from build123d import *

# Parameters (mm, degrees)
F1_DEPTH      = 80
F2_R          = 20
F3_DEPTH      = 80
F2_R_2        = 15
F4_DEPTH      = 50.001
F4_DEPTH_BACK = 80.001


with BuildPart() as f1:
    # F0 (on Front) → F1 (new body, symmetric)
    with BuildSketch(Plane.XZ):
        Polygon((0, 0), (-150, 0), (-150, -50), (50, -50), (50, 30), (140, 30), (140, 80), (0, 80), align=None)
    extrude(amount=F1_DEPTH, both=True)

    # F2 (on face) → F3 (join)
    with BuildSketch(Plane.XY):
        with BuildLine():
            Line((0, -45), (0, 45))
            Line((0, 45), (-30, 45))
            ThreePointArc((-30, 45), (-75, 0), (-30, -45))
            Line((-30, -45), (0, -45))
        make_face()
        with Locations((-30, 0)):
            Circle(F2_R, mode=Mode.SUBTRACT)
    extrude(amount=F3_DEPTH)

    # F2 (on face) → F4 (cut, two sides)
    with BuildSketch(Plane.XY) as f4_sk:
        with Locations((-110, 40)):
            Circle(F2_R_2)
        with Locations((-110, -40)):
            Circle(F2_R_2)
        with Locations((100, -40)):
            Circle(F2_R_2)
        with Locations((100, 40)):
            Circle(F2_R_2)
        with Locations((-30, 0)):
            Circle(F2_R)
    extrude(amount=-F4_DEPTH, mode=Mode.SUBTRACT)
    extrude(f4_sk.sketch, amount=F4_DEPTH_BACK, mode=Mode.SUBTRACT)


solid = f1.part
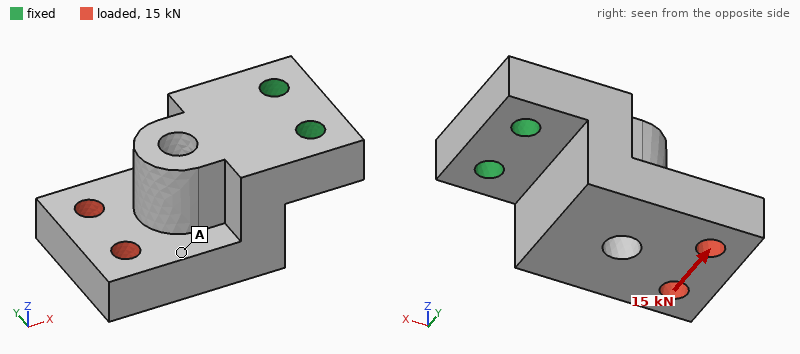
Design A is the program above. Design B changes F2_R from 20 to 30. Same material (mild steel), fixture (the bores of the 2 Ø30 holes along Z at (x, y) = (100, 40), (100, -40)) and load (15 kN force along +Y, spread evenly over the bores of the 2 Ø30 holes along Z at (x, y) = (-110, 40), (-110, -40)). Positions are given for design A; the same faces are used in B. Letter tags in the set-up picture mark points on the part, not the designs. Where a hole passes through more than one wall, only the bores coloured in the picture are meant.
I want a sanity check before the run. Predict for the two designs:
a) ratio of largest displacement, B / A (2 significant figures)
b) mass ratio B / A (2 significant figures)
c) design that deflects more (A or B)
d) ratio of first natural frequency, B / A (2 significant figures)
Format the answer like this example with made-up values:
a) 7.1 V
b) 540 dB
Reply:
a) 1.1
b) 0.93
c) B
d) 1.0
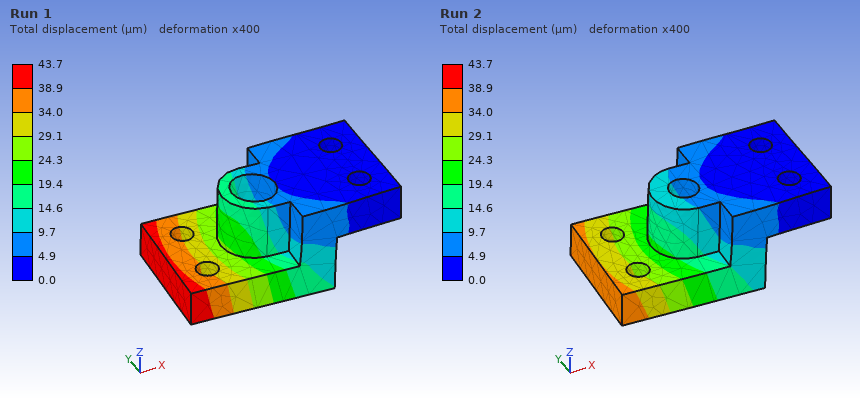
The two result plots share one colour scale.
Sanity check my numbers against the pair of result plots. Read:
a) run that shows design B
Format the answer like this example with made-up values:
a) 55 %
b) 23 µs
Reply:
a) Run 1
